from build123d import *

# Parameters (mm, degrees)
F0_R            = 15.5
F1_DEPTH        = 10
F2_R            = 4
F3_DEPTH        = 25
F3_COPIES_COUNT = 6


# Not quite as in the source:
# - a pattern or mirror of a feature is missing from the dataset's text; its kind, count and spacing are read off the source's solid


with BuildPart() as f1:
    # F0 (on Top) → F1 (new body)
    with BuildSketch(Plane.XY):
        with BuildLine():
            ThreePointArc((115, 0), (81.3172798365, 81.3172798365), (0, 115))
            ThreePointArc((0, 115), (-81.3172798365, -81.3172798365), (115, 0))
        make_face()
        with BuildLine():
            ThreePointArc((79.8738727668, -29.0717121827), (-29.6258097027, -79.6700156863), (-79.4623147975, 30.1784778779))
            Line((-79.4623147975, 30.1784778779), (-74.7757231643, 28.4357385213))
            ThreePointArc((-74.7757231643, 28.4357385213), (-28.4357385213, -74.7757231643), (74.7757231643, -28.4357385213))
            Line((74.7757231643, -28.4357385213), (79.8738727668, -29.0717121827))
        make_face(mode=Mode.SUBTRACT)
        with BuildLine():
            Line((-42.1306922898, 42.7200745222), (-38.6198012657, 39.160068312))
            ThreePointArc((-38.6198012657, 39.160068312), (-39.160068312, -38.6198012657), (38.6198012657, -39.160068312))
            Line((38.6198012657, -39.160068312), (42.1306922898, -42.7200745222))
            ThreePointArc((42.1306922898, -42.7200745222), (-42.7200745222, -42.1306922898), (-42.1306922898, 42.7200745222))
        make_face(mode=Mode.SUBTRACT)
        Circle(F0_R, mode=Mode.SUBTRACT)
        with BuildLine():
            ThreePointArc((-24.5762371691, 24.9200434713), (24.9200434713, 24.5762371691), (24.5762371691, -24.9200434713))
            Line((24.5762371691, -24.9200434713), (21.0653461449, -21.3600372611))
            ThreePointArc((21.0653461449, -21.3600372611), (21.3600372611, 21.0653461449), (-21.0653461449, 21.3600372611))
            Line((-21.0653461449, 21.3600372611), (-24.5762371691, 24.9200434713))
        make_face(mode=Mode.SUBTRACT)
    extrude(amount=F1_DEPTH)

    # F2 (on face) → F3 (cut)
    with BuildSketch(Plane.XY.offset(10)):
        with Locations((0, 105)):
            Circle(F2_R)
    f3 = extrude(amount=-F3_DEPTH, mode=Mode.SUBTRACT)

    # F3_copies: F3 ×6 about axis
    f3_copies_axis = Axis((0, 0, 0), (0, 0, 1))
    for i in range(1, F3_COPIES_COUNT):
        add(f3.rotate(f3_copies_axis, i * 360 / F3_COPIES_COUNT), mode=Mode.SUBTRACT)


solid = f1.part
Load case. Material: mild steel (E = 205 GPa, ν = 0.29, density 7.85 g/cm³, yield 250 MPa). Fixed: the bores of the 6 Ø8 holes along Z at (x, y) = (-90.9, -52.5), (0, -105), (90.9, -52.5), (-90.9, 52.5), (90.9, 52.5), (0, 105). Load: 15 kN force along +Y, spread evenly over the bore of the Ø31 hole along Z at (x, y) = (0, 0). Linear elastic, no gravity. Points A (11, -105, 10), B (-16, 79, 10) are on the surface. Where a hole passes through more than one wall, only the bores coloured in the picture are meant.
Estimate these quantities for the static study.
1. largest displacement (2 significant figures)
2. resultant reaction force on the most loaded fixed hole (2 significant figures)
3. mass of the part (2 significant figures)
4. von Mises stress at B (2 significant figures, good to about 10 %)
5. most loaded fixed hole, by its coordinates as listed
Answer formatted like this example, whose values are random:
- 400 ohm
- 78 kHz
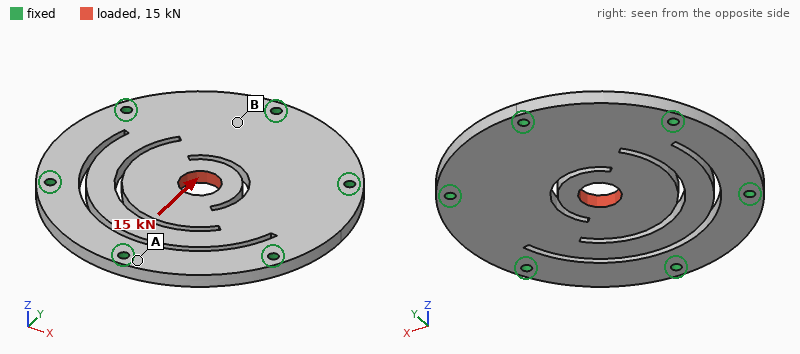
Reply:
- 32 µm
- 7.0 kN
- 3.0 kg
- 21 MPa
- (0, 105)
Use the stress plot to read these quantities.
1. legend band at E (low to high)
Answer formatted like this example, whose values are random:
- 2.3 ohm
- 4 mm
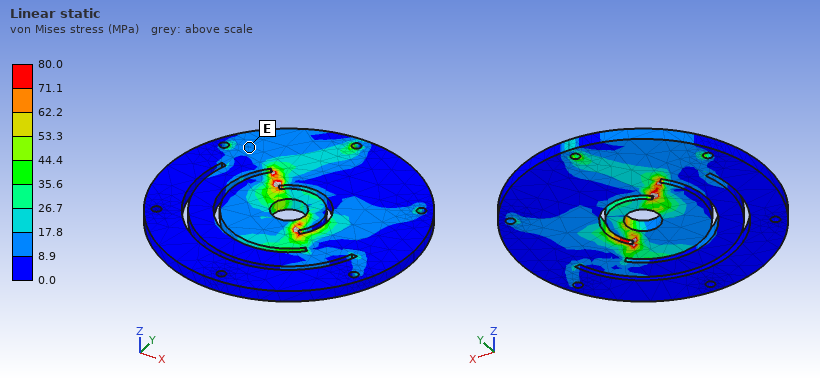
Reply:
- 8.9 to 17.8 MPa
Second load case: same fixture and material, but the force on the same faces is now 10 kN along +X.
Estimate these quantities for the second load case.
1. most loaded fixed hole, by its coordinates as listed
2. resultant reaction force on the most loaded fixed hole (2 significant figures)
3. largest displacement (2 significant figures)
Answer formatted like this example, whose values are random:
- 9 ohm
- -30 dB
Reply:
- (90.9, 52.5)
- 3.5 kN
- 23 µm
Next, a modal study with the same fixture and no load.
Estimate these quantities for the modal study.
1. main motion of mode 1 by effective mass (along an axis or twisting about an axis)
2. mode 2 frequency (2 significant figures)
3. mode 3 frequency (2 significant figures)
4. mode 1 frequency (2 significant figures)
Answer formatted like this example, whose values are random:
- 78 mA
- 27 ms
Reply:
- along Z
- 1000 Hz
- 1800 Hz
- 590 Hz
